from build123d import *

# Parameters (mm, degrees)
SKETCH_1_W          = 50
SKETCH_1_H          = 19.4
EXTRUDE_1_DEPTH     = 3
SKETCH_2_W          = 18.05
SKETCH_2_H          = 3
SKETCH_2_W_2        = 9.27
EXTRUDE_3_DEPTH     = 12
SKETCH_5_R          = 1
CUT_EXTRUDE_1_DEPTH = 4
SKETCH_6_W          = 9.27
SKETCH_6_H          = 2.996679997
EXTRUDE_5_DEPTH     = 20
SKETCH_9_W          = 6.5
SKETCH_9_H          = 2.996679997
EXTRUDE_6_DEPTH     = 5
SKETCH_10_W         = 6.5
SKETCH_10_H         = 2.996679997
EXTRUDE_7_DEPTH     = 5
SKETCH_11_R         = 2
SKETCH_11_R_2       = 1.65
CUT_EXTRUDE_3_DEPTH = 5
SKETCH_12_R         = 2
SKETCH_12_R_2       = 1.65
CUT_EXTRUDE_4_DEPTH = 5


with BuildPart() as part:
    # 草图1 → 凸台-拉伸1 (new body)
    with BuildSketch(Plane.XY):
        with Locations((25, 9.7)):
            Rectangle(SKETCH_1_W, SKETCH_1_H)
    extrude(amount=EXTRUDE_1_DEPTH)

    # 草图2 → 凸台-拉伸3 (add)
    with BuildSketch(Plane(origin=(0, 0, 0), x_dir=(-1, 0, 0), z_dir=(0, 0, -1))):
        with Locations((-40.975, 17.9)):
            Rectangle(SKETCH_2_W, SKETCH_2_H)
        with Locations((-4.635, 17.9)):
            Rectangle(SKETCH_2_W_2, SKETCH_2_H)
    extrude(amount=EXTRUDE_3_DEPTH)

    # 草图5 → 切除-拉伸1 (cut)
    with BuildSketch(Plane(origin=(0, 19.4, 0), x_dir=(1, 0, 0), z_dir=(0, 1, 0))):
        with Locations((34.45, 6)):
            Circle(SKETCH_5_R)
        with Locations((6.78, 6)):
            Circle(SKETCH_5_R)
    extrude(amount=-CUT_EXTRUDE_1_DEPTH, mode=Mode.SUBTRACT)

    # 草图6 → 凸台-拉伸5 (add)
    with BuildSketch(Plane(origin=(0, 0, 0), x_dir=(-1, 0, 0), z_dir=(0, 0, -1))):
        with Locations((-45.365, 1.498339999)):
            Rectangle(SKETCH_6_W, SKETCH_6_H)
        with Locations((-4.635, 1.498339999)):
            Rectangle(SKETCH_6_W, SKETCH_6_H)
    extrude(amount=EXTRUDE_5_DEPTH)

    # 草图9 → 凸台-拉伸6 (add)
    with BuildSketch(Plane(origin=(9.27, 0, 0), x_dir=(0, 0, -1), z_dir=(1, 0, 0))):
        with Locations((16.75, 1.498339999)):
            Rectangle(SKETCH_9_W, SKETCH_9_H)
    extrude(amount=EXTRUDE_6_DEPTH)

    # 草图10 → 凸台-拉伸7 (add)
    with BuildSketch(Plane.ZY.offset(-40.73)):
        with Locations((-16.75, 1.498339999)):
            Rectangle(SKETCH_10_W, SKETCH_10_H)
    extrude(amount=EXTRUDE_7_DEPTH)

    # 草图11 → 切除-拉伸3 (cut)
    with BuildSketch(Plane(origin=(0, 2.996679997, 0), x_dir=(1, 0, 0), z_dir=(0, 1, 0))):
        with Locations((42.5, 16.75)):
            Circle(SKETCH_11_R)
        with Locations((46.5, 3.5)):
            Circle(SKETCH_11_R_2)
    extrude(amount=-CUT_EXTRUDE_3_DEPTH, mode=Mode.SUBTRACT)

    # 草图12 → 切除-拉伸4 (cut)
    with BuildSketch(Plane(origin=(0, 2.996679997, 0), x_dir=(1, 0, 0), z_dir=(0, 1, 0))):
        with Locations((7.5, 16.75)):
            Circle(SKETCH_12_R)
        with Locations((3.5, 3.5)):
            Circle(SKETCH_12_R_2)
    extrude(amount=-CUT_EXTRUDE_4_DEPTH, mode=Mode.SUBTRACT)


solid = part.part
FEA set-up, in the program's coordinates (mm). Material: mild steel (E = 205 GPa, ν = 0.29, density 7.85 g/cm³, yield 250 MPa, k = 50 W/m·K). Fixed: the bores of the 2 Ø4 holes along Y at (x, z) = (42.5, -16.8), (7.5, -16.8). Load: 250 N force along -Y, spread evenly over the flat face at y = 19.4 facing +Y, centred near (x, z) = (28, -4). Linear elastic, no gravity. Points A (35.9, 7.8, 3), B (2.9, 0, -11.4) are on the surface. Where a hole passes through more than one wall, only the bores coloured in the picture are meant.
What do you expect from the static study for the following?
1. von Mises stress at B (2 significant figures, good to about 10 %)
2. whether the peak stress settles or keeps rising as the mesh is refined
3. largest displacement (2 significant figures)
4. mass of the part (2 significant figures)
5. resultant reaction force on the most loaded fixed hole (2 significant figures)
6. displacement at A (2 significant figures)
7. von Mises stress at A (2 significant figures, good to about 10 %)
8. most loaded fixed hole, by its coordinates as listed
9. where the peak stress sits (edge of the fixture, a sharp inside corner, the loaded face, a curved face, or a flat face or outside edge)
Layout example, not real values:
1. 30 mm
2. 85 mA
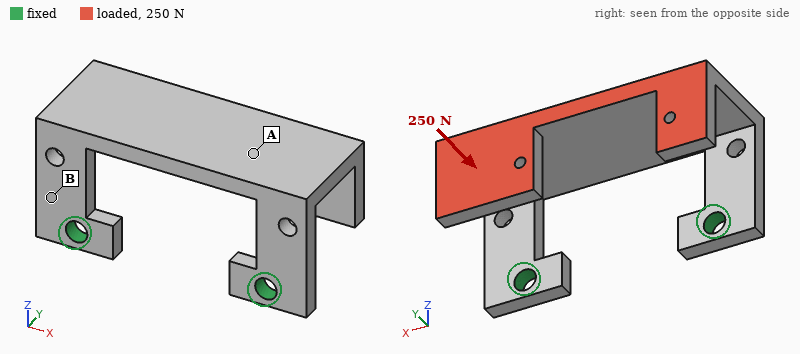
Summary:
1. 54 MPa
2. keeps rising
3. 40 µm
4. 40 g
5. 140 N
6. 35 µm
7. 15 MPa
8. (42.5, -16.8)
9. edge of the fixture
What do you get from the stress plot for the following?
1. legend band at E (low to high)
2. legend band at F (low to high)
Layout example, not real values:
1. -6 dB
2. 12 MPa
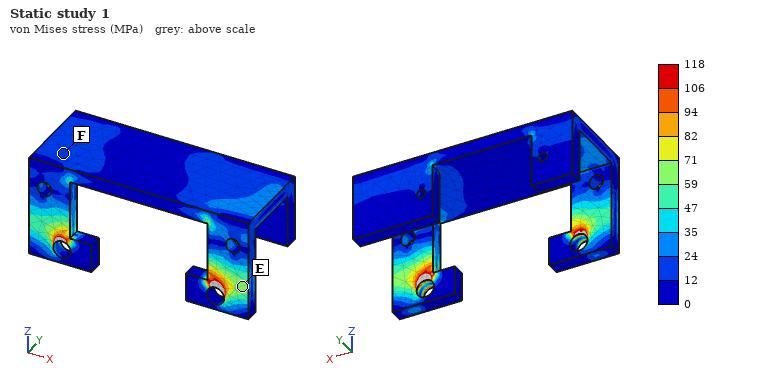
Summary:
1. 59 to 71 MPa
2. 12 to 24 MPa
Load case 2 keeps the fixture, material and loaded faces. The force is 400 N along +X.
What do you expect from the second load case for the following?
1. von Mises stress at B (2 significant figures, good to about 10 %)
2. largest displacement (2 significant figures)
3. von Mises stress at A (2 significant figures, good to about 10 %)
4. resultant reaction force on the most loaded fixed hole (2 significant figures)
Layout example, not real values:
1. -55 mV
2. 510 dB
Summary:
1. 94 MPa
2. 85 µm
3. 36 MPa
4. 260 N
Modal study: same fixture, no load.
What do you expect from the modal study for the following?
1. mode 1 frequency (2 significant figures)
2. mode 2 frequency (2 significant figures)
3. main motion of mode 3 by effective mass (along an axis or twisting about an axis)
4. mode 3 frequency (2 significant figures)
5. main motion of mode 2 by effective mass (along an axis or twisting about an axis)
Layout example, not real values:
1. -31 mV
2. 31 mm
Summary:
1. 1300 Hz
2. 2600 Hz
3. along Y
4. 3300 Hz
5. along X
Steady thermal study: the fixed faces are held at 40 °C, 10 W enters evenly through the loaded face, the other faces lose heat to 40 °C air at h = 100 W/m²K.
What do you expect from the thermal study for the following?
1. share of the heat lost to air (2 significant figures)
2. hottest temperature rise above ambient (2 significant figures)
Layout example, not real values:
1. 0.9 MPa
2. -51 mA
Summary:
1. 78 %
2. 42 K
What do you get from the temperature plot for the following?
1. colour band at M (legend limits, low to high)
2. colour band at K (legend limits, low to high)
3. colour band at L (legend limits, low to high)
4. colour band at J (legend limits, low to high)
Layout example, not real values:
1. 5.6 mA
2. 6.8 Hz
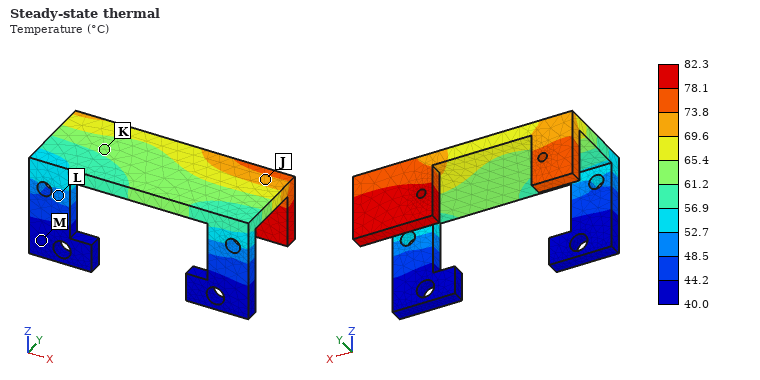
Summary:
1. 40.0 to 44.2 °C
2. 61.2 to 65.4 °C
3. 48.5 to 52.7 °C
4. 69.6 to 73.8 °C
